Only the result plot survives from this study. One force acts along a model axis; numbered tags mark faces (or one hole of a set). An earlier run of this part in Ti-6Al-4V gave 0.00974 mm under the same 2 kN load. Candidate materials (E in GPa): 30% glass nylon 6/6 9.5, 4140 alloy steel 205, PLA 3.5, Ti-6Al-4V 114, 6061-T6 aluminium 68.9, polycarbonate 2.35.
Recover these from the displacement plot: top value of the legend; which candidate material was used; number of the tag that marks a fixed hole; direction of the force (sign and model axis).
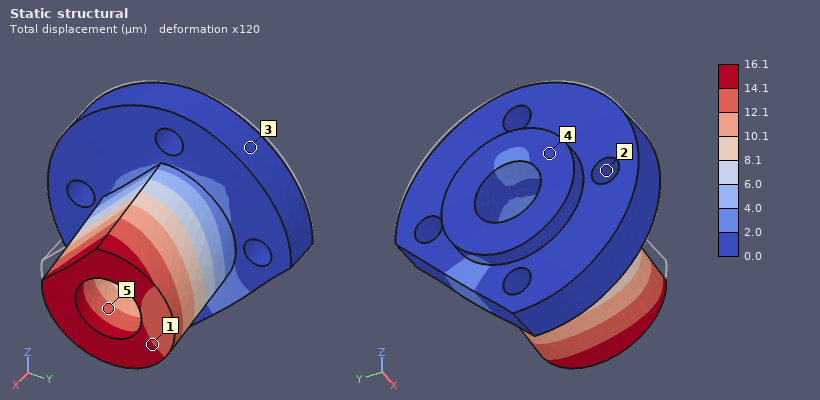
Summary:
16.1 µm
6061-T6 aluminium
2
-Z
